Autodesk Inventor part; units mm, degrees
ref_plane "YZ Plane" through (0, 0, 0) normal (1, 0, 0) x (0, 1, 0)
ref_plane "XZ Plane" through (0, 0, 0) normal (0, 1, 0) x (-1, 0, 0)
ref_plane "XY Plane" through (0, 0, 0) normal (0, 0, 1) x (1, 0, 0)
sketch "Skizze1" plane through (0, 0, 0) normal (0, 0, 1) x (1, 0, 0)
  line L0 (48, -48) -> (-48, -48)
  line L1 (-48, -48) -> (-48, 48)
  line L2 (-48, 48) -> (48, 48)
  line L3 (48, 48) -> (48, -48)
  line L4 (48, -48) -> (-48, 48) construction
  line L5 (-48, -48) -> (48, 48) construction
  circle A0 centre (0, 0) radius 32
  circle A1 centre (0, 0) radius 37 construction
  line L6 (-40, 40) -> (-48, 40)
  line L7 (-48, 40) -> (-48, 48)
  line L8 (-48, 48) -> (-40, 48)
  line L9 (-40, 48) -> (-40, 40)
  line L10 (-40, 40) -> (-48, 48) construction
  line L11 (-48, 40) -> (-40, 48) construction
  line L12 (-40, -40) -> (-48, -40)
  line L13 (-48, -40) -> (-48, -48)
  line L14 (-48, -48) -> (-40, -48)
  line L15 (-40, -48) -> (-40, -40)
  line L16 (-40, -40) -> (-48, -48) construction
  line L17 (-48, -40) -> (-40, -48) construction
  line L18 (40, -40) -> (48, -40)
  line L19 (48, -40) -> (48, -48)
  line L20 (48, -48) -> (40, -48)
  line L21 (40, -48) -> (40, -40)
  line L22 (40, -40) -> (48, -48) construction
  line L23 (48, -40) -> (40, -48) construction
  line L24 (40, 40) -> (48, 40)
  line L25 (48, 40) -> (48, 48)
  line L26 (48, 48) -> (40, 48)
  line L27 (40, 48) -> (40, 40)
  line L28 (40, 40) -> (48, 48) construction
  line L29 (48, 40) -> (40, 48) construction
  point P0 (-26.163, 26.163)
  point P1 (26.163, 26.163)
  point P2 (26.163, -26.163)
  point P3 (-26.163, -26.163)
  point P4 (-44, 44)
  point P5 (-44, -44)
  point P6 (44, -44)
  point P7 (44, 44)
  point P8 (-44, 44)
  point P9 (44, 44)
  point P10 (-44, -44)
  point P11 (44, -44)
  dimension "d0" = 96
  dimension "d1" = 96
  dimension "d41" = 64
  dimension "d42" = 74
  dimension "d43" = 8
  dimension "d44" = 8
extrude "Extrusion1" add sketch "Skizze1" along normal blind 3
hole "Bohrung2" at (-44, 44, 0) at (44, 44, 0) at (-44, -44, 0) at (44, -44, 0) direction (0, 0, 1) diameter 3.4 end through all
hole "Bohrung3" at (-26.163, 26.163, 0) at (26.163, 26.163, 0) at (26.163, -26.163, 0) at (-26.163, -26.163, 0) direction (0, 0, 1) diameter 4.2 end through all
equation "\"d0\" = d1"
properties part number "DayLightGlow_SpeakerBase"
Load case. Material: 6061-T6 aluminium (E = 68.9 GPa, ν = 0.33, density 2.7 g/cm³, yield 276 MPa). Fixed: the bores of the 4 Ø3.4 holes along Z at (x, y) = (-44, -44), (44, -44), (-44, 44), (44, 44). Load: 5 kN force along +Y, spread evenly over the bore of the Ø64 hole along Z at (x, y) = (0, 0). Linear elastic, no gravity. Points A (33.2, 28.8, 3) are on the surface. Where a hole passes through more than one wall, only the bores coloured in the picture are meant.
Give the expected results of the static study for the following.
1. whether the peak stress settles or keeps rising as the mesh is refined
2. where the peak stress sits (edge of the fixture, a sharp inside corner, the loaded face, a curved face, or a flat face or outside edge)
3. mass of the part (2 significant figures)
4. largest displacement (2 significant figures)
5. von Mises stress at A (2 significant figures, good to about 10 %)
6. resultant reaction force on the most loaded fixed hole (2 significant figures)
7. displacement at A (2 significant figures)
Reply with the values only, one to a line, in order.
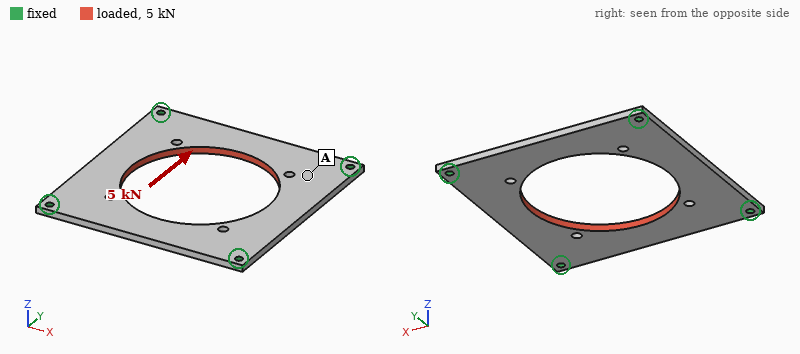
keeps rising
edge of the fixture
48 g
40 µm
13 MPa
1.4 kN
15 µm
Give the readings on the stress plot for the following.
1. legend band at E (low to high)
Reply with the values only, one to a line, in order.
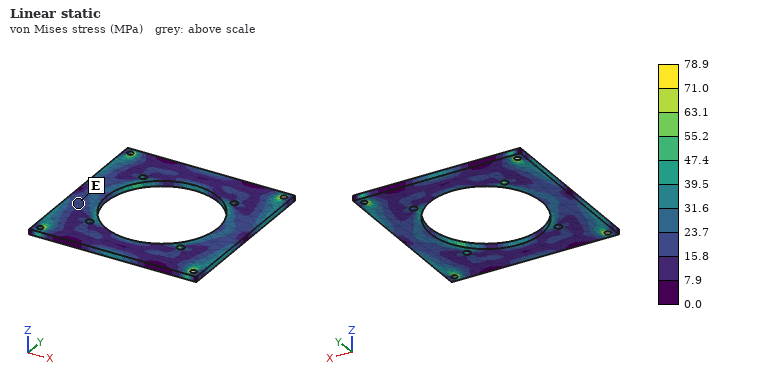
15.8 to 23.7 MPa
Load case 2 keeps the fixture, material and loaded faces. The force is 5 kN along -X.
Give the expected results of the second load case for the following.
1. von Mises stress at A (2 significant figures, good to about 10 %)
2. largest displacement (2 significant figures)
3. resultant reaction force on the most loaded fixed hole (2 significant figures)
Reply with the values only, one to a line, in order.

16 MPa
40 µm
1.4 kN
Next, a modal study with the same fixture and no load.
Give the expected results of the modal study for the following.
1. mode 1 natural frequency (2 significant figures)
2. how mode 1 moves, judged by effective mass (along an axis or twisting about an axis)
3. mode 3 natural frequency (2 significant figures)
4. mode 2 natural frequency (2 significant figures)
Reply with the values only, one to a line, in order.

1600 Hz
along Z
2100 Hz
2100 Hz
